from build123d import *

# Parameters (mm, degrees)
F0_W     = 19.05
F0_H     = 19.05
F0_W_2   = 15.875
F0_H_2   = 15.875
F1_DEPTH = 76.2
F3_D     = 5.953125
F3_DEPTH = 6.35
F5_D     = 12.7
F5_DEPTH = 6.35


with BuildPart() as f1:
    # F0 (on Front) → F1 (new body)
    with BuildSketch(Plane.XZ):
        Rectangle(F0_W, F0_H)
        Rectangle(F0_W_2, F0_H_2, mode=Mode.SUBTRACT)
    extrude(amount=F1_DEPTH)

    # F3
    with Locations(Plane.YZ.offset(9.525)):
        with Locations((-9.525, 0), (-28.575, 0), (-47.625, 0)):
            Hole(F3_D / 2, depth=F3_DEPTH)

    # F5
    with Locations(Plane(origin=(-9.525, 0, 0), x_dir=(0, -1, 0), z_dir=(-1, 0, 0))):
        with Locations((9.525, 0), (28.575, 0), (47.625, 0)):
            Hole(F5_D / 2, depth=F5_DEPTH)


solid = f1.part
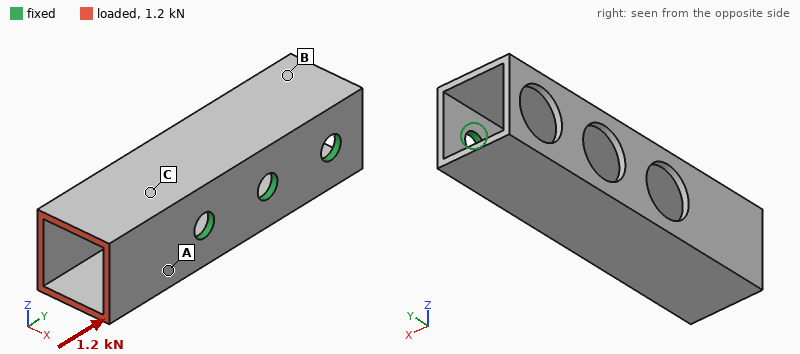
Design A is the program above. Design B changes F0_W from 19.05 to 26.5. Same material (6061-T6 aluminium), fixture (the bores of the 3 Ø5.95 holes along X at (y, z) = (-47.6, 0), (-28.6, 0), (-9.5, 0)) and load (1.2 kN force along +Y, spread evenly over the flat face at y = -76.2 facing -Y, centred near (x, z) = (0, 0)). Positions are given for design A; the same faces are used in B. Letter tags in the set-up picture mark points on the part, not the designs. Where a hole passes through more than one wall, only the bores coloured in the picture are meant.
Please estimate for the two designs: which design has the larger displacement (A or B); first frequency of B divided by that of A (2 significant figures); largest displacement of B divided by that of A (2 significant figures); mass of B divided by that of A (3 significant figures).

A
1.3
0.23
2.18
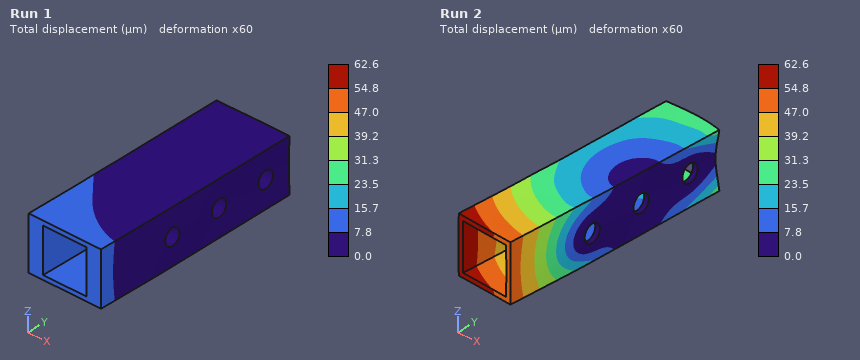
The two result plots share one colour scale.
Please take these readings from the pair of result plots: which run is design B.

Run 1
